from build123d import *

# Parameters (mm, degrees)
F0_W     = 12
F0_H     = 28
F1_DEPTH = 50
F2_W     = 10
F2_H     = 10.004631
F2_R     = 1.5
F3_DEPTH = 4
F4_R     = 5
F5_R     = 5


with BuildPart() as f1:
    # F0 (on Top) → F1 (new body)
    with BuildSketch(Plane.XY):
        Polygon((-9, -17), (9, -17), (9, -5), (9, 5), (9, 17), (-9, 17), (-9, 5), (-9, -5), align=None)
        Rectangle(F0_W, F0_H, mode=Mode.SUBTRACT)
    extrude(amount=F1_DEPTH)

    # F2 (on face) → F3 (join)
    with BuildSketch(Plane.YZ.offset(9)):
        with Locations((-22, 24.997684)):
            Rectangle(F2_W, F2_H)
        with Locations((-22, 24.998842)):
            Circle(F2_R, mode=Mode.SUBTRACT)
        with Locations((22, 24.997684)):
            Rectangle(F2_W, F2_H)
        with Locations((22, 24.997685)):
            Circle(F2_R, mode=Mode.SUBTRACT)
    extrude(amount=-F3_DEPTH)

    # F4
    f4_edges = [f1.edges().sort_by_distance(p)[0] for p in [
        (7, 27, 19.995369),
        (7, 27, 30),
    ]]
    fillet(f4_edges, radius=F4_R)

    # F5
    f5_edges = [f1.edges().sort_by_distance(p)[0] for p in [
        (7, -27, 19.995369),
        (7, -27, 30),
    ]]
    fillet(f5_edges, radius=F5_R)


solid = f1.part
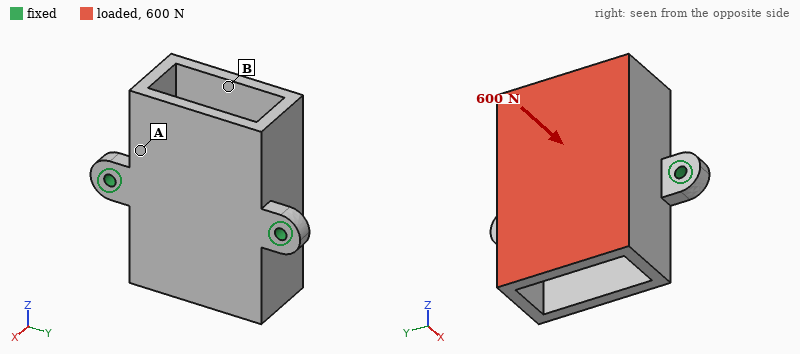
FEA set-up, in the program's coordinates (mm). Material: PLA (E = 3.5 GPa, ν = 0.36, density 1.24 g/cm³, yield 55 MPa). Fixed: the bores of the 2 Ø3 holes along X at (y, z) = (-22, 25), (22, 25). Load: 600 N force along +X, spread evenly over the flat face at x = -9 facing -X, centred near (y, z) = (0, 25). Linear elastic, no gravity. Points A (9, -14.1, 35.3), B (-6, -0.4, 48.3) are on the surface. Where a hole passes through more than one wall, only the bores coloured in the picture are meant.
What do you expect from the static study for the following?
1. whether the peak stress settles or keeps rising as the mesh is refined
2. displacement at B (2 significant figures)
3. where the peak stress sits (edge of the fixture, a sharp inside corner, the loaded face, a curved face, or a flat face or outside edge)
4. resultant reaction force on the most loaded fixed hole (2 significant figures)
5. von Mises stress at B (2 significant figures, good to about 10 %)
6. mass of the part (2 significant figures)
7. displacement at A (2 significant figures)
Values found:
keeps rising
0.31 mm
edge of the fixture
310 N
10 MPa
18 g
0.11 mm
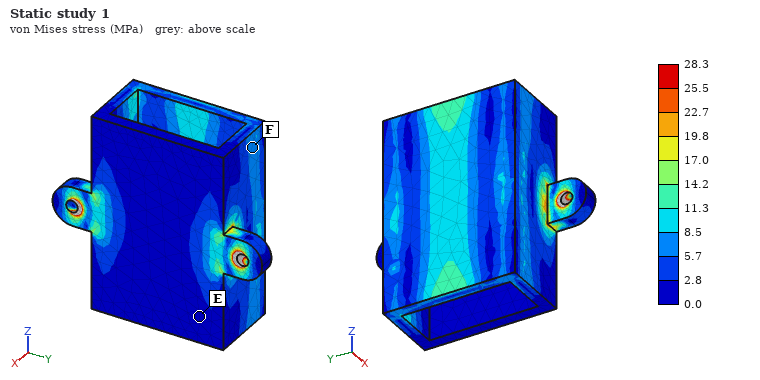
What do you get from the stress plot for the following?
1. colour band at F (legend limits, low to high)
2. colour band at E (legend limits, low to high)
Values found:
5.7 to 8.5 MPa
0.0 to 2.8 MPa
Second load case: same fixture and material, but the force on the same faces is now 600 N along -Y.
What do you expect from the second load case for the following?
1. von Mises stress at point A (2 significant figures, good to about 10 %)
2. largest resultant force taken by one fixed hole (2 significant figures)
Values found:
12 MPa
380 N
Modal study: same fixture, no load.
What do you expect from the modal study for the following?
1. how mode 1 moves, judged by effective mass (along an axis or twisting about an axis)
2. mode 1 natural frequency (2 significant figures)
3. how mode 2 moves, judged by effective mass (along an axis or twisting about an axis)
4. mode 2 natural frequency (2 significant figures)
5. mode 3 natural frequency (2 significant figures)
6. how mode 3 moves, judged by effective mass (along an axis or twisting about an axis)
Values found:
along Z
640 Hz
along Y
2100 Hz
2400 Hz
twisting about X
